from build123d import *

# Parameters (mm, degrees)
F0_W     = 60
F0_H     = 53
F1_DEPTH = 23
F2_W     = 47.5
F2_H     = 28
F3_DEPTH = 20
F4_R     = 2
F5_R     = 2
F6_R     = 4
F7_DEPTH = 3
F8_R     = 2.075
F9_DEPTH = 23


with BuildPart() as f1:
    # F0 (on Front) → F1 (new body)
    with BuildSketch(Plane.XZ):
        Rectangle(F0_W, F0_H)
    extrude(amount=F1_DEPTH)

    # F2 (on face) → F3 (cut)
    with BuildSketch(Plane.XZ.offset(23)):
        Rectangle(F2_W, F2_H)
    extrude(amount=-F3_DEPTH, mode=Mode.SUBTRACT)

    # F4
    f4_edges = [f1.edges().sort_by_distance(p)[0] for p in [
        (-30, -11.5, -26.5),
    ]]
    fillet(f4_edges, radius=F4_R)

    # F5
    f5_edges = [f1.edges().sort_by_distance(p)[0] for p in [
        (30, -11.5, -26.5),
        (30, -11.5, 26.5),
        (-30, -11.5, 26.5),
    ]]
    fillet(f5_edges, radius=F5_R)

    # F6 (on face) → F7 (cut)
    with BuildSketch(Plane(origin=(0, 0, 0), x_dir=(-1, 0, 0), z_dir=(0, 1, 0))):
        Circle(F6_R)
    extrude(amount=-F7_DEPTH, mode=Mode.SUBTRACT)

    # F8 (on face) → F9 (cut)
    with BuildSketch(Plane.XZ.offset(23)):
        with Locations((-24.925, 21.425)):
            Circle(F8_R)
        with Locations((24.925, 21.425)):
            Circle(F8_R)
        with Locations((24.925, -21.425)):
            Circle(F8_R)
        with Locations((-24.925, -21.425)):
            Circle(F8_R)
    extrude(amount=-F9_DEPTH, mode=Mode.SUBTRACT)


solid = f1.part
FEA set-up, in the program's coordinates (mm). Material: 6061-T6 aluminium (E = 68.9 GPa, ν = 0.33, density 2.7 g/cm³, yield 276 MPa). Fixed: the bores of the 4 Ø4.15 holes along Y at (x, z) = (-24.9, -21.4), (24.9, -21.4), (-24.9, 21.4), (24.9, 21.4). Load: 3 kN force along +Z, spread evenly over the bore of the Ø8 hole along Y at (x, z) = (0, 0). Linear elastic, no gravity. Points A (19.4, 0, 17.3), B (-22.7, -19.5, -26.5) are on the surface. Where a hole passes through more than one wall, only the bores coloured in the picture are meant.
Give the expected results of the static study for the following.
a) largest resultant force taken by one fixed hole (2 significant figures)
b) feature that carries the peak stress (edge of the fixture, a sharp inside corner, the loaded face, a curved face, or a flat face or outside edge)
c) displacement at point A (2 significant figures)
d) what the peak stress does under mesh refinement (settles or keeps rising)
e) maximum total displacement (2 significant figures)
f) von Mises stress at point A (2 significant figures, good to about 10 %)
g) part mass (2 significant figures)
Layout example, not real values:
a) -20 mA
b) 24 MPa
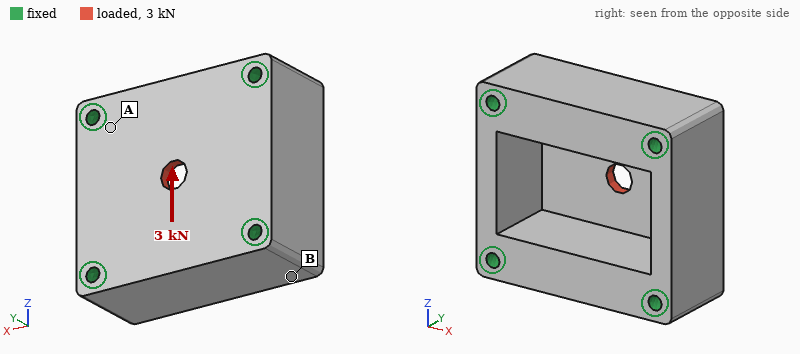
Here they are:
a) 870 N
b) a sharp inside corner
c) 1.5 µm
d) keeps rising
e) 10 µm
f) 15 MPa
g) 120 g
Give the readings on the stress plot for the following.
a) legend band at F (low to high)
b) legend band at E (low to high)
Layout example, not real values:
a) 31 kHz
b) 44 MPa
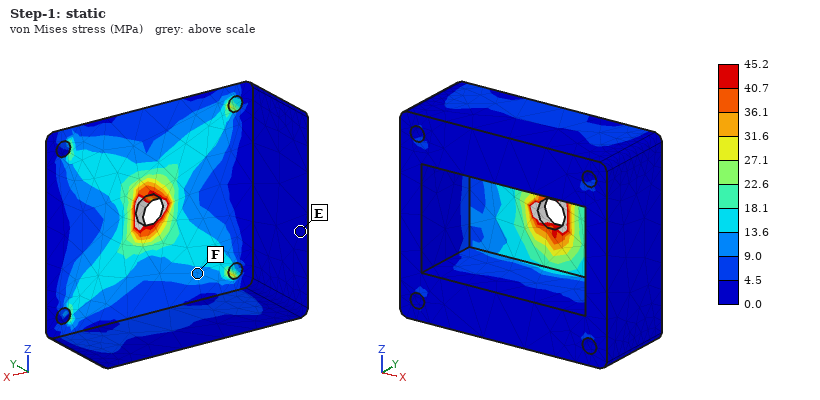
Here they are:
a) 9.0 to 13.6 MPa
b) 0.0 to 4.5 MPa
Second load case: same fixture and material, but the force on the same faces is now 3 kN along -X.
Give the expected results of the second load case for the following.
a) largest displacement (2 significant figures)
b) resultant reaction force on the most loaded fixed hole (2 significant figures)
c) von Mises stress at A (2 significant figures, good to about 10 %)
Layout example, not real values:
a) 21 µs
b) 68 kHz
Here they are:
a) 8.7 µm
b) 840 N
c) 10 MPa
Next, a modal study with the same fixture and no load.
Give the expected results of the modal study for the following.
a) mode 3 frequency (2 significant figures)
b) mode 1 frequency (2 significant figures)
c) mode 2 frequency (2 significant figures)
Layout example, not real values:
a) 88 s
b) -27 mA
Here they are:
a) 20 kHz
b) 17 kHz
c) 20 kHz
